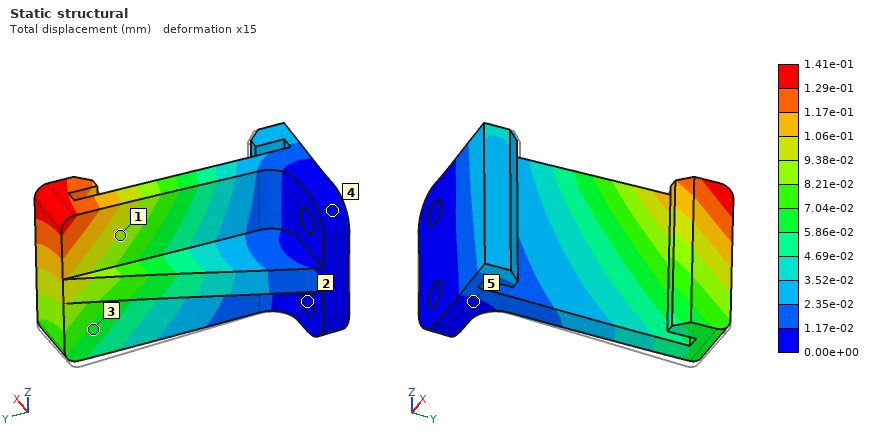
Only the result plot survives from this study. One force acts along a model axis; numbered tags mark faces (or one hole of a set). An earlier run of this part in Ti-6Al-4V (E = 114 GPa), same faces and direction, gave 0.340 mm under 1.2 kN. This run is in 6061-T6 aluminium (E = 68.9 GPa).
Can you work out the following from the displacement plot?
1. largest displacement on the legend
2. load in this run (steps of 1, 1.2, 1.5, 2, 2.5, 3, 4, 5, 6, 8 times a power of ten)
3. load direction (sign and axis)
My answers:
1.41e-01 mm
300 N
+X
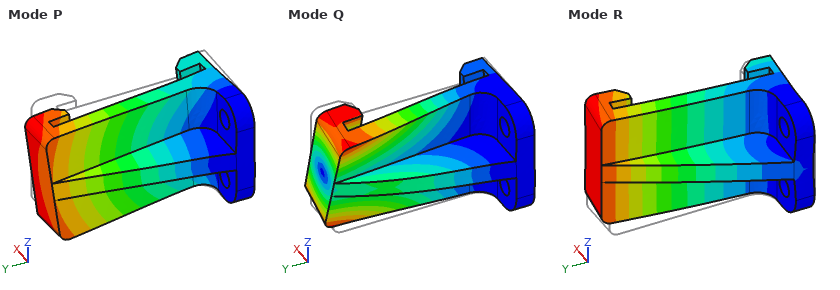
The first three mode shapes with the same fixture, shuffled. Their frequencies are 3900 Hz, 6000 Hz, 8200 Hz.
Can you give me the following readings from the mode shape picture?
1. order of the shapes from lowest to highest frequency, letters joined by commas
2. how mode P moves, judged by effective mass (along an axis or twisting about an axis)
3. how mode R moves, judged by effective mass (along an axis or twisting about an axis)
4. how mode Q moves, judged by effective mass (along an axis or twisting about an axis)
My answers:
R, P, Q
along Z
along X
twisting about Y
